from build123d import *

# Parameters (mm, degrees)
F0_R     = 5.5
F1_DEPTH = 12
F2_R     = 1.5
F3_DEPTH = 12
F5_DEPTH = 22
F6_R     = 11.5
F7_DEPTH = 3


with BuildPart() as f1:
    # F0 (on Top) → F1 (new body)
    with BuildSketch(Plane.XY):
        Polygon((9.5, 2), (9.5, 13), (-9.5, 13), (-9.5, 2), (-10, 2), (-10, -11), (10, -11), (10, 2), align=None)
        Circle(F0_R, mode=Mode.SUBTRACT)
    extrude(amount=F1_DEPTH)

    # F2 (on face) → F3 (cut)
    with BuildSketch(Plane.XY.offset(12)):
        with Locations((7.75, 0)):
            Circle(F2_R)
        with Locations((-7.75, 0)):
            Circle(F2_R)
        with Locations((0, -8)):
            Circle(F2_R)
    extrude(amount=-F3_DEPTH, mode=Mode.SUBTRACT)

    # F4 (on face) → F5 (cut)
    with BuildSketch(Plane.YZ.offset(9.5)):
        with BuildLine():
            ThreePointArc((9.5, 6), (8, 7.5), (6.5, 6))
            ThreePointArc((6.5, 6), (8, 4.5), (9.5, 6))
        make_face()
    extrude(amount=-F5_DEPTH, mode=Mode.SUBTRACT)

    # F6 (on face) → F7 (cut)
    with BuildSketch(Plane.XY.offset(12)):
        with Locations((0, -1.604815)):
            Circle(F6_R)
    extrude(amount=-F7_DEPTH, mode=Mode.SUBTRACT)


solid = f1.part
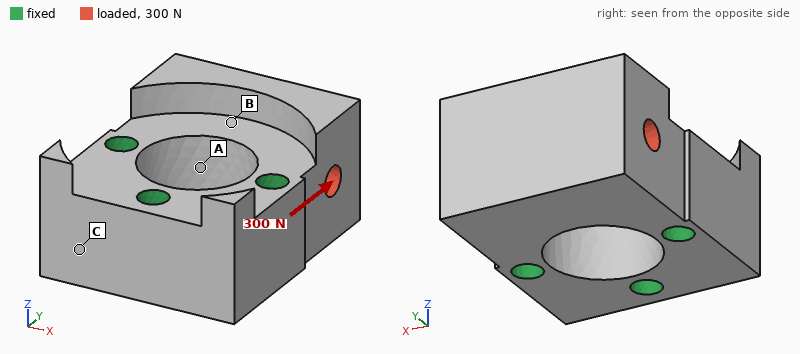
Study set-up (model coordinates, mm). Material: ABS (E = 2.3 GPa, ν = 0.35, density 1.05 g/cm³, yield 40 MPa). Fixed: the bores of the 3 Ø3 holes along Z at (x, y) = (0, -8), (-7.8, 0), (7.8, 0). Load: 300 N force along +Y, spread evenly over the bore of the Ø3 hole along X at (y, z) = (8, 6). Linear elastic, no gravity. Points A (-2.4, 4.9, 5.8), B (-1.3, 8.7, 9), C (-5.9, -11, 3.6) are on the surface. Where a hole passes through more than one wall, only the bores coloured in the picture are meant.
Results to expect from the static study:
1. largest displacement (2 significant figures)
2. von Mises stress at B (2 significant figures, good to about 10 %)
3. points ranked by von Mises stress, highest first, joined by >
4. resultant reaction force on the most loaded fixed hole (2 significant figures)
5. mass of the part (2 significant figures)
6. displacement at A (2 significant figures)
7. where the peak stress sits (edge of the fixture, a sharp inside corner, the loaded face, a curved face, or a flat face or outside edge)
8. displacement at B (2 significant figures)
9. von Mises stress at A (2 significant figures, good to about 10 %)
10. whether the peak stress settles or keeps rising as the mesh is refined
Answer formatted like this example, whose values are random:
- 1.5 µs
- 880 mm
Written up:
- 37 µm
- 1.7 MPa
- A > B > C
- 160 N
- 3.5 g
- 18 µm
- edge of the fixture
- 28 µm
- 3.2 MPa
- keeps rising
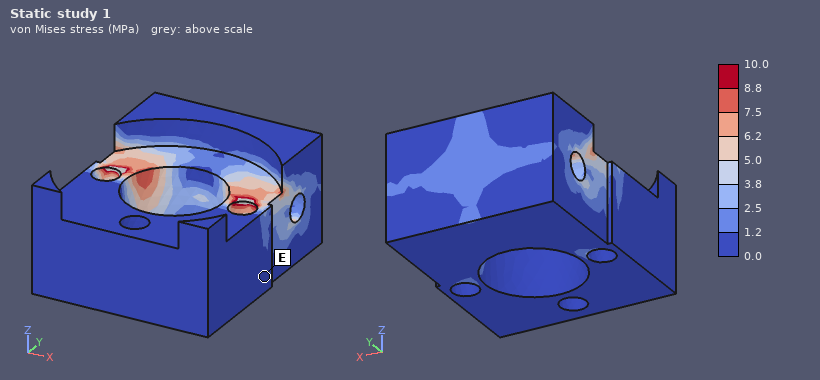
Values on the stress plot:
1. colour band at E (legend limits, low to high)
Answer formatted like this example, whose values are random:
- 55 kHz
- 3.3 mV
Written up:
- 0.0 to 1.2 MPa
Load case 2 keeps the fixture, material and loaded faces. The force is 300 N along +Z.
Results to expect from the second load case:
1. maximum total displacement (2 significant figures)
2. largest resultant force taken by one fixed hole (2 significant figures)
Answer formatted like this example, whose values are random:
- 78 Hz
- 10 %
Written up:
- 0.10 mm
- 150 N
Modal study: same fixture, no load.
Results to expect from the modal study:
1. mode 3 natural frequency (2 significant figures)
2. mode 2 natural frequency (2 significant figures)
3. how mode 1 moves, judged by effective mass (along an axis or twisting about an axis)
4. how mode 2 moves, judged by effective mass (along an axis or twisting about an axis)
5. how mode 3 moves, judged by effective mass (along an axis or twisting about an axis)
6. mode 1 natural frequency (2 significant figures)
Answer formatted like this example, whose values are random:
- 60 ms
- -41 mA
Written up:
- 11 kHz
- 9600 Hz
- along Z
- along X
- along X
- 6800 Hz
